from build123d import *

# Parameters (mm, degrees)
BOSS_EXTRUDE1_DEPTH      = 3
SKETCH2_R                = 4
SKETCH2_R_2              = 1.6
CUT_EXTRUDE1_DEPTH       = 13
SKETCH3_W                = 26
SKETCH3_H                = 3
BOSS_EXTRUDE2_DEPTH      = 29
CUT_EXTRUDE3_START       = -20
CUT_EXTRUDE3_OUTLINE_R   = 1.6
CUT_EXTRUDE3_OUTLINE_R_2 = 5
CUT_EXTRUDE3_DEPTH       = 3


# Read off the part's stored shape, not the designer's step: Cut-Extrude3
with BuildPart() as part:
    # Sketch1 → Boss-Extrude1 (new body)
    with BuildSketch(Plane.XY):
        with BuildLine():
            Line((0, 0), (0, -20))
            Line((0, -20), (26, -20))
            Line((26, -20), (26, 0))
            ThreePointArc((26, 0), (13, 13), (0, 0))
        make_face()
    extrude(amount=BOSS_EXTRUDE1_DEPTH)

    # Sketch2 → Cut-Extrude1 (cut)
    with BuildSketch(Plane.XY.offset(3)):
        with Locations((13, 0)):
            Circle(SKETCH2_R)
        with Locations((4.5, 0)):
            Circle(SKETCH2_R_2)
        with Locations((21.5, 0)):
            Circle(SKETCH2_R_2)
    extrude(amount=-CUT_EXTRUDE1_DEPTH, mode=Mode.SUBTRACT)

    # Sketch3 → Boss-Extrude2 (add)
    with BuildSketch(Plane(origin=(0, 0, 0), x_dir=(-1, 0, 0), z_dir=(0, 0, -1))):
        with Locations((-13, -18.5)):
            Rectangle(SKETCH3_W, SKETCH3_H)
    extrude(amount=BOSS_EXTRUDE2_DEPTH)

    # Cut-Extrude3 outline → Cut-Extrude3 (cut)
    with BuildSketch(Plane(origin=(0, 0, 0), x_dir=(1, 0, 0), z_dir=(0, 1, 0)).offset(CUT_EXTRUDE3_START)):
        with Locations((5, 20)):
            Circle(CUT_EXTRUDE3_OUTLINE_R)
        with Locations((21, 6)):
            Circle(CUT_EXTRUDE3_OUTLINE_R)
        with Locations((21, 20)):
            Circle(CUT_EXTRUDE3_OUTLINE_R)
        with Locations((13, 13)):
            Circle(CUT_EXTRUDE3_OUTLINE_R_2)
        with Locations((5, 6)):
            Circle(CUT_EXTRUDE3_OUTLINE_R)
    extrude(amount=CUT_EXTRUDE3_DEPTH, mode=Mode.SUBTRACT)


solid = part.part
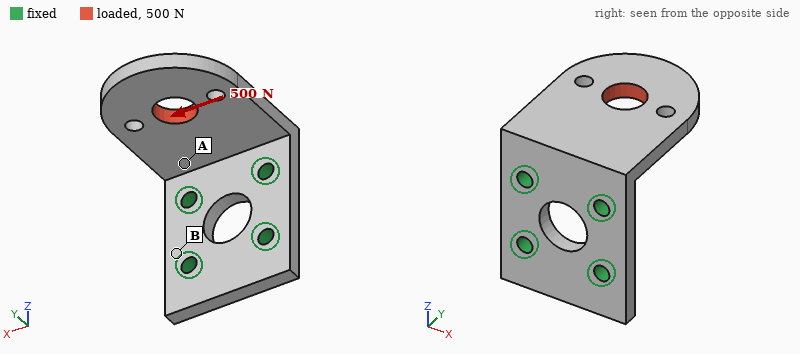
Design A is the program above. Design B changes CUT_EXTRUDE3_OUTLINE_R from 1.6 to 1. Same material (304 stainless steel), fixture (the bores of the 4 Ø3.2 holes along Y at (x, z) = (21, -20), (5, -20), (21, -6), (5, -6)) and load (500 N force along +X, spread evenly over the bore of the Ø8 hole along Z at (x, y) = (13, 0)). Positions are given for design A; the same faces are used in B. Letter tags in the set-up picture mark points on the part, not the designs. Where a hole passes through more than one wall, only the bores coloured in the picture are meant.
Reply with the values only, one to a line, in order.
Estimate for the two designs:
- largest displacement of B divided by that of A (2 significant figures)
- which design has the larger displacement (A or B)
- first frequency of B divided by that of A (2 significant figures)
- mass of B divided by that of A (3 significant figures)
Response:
1.2
B
0.96
1.01
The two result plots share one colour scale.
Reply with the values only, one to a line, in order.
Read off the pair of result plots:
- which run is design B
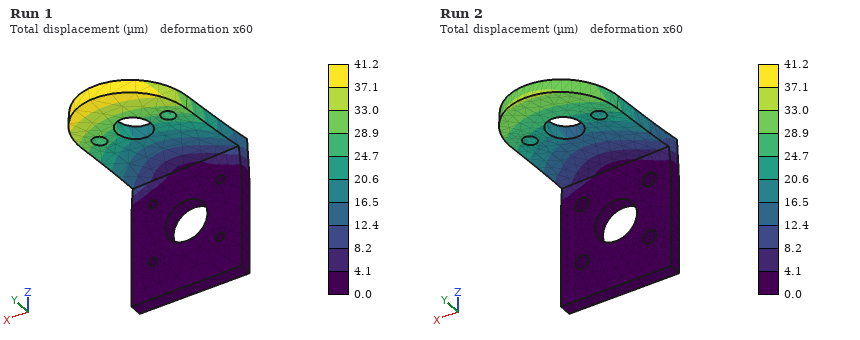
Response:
Run 1
